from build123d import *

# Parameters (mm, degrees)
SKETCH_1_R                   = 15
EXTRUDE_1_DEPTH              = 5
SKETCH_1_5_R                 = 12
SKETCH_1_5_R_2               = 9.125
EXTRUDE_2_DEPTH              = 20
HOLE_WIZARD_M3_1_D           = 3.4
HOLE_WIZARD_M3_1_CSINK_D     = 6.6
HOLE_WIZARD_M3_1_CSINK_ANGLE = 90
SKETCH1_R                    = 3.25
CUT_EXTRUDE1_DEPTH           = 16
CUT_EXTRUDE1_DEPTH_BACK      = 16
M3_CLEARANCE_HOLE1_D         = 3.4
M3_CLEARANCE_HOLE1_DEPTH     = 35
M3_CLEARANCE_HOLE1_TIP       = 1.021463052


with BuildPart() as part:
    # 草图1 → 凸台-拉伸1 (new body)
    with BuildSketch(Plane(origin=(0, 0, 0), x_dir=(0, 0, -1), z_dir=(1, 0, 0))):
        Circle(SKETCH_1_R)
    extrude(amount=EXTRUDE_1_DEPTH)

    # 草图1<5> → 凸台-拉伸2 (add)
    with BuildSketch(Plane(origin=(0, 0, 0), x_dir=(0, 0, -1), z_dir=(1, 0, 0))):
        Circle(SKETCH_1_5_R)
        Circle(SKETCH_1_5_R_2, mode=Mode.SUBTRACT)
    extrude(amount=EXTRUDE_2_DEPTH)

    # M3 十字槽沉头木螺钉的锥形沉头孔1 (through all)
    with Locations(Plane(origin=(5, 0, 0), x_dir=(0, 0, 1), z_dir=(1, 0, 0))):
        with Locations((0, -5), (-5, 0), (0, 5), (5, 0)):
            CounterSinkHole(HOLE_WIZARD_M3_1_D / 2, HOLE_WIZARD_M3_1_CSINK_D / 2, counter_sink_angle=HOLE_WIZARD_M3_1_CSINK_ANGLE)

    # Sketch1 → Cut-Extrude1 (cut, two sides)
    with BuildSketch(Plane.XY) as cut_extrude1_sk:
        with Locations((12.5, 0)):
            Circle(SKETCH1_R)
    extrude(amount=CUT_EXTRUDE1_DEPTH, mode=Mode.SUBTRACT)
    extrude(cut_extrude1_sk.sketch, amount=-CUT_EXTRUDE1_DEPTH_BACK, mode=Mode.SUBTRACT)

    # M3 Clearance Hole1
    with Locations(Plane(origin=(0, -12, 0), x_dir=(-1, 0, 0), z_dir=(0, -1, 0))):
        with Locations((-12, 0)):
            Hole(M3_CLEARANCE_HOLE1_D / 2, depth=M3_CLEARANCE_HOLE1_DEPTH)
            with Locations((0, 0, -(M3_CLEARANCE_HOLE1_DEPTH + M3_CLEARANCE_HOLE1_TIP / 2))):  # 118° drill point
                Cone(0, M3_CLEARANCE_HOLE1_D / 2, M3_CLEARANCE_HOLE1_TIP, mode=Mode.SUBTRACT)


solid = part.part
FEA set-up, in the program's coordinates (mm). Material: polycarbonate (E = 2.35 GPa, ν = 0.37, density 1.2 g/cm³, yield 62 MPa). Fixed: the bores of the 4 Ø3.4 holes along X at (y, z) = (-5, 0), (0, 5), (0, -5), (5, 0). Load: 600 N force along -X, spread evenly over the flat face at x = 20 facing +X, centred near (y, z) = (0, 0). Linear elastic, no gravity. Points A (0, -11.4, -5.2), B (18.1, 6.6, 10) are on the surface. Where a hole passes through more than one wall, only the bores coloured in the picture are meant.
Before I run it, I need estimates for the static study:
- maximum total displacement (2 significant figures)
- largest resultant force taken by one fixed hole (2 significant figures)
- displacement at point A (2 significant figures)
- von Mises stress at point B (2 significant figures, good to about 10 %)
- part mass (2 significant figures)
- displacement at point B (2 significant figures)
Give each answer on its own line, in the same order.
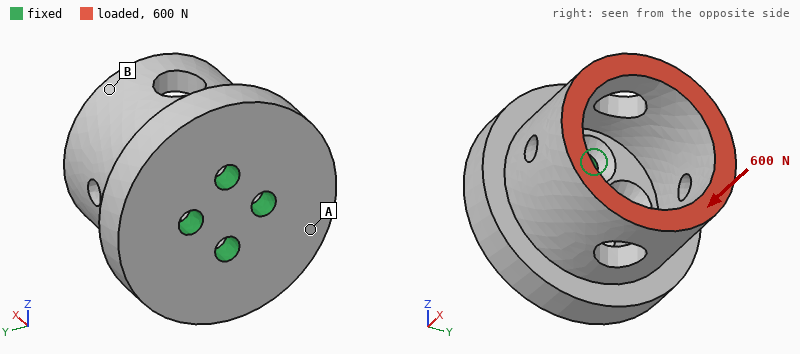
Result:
76 µm
160 N
41 µm
3.8 MPa
7.1 g
57 µm
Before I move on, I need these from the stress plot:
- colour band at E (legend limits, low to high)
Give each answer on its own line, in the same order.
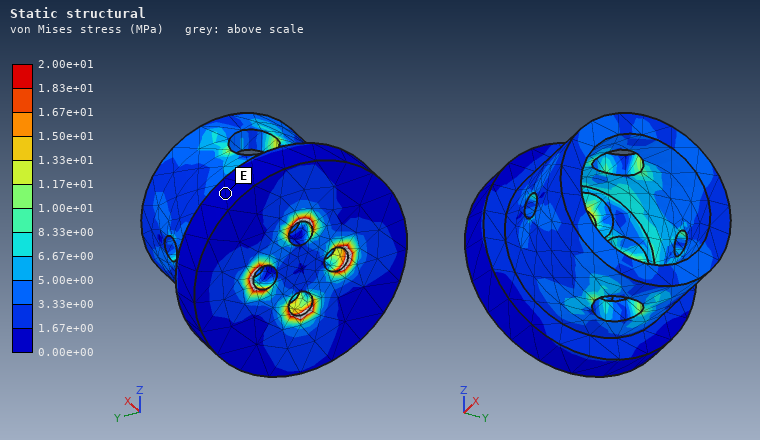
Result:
0.00e+00 to 1.67e+00 MPa
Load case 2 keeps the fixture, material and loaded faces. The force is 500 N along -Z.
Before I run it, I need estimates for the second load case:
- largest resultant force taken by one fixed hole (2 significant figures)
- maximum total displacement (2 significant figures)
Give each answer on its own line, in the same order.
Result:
490 N
0.51 mm
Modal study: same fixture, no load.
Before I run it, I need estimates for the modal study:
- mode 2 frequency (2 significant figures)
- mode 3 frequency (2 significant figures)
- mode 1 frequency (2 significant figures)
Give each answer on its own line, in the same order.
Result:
4100 Hz
5500 Hz
4000 Hz
